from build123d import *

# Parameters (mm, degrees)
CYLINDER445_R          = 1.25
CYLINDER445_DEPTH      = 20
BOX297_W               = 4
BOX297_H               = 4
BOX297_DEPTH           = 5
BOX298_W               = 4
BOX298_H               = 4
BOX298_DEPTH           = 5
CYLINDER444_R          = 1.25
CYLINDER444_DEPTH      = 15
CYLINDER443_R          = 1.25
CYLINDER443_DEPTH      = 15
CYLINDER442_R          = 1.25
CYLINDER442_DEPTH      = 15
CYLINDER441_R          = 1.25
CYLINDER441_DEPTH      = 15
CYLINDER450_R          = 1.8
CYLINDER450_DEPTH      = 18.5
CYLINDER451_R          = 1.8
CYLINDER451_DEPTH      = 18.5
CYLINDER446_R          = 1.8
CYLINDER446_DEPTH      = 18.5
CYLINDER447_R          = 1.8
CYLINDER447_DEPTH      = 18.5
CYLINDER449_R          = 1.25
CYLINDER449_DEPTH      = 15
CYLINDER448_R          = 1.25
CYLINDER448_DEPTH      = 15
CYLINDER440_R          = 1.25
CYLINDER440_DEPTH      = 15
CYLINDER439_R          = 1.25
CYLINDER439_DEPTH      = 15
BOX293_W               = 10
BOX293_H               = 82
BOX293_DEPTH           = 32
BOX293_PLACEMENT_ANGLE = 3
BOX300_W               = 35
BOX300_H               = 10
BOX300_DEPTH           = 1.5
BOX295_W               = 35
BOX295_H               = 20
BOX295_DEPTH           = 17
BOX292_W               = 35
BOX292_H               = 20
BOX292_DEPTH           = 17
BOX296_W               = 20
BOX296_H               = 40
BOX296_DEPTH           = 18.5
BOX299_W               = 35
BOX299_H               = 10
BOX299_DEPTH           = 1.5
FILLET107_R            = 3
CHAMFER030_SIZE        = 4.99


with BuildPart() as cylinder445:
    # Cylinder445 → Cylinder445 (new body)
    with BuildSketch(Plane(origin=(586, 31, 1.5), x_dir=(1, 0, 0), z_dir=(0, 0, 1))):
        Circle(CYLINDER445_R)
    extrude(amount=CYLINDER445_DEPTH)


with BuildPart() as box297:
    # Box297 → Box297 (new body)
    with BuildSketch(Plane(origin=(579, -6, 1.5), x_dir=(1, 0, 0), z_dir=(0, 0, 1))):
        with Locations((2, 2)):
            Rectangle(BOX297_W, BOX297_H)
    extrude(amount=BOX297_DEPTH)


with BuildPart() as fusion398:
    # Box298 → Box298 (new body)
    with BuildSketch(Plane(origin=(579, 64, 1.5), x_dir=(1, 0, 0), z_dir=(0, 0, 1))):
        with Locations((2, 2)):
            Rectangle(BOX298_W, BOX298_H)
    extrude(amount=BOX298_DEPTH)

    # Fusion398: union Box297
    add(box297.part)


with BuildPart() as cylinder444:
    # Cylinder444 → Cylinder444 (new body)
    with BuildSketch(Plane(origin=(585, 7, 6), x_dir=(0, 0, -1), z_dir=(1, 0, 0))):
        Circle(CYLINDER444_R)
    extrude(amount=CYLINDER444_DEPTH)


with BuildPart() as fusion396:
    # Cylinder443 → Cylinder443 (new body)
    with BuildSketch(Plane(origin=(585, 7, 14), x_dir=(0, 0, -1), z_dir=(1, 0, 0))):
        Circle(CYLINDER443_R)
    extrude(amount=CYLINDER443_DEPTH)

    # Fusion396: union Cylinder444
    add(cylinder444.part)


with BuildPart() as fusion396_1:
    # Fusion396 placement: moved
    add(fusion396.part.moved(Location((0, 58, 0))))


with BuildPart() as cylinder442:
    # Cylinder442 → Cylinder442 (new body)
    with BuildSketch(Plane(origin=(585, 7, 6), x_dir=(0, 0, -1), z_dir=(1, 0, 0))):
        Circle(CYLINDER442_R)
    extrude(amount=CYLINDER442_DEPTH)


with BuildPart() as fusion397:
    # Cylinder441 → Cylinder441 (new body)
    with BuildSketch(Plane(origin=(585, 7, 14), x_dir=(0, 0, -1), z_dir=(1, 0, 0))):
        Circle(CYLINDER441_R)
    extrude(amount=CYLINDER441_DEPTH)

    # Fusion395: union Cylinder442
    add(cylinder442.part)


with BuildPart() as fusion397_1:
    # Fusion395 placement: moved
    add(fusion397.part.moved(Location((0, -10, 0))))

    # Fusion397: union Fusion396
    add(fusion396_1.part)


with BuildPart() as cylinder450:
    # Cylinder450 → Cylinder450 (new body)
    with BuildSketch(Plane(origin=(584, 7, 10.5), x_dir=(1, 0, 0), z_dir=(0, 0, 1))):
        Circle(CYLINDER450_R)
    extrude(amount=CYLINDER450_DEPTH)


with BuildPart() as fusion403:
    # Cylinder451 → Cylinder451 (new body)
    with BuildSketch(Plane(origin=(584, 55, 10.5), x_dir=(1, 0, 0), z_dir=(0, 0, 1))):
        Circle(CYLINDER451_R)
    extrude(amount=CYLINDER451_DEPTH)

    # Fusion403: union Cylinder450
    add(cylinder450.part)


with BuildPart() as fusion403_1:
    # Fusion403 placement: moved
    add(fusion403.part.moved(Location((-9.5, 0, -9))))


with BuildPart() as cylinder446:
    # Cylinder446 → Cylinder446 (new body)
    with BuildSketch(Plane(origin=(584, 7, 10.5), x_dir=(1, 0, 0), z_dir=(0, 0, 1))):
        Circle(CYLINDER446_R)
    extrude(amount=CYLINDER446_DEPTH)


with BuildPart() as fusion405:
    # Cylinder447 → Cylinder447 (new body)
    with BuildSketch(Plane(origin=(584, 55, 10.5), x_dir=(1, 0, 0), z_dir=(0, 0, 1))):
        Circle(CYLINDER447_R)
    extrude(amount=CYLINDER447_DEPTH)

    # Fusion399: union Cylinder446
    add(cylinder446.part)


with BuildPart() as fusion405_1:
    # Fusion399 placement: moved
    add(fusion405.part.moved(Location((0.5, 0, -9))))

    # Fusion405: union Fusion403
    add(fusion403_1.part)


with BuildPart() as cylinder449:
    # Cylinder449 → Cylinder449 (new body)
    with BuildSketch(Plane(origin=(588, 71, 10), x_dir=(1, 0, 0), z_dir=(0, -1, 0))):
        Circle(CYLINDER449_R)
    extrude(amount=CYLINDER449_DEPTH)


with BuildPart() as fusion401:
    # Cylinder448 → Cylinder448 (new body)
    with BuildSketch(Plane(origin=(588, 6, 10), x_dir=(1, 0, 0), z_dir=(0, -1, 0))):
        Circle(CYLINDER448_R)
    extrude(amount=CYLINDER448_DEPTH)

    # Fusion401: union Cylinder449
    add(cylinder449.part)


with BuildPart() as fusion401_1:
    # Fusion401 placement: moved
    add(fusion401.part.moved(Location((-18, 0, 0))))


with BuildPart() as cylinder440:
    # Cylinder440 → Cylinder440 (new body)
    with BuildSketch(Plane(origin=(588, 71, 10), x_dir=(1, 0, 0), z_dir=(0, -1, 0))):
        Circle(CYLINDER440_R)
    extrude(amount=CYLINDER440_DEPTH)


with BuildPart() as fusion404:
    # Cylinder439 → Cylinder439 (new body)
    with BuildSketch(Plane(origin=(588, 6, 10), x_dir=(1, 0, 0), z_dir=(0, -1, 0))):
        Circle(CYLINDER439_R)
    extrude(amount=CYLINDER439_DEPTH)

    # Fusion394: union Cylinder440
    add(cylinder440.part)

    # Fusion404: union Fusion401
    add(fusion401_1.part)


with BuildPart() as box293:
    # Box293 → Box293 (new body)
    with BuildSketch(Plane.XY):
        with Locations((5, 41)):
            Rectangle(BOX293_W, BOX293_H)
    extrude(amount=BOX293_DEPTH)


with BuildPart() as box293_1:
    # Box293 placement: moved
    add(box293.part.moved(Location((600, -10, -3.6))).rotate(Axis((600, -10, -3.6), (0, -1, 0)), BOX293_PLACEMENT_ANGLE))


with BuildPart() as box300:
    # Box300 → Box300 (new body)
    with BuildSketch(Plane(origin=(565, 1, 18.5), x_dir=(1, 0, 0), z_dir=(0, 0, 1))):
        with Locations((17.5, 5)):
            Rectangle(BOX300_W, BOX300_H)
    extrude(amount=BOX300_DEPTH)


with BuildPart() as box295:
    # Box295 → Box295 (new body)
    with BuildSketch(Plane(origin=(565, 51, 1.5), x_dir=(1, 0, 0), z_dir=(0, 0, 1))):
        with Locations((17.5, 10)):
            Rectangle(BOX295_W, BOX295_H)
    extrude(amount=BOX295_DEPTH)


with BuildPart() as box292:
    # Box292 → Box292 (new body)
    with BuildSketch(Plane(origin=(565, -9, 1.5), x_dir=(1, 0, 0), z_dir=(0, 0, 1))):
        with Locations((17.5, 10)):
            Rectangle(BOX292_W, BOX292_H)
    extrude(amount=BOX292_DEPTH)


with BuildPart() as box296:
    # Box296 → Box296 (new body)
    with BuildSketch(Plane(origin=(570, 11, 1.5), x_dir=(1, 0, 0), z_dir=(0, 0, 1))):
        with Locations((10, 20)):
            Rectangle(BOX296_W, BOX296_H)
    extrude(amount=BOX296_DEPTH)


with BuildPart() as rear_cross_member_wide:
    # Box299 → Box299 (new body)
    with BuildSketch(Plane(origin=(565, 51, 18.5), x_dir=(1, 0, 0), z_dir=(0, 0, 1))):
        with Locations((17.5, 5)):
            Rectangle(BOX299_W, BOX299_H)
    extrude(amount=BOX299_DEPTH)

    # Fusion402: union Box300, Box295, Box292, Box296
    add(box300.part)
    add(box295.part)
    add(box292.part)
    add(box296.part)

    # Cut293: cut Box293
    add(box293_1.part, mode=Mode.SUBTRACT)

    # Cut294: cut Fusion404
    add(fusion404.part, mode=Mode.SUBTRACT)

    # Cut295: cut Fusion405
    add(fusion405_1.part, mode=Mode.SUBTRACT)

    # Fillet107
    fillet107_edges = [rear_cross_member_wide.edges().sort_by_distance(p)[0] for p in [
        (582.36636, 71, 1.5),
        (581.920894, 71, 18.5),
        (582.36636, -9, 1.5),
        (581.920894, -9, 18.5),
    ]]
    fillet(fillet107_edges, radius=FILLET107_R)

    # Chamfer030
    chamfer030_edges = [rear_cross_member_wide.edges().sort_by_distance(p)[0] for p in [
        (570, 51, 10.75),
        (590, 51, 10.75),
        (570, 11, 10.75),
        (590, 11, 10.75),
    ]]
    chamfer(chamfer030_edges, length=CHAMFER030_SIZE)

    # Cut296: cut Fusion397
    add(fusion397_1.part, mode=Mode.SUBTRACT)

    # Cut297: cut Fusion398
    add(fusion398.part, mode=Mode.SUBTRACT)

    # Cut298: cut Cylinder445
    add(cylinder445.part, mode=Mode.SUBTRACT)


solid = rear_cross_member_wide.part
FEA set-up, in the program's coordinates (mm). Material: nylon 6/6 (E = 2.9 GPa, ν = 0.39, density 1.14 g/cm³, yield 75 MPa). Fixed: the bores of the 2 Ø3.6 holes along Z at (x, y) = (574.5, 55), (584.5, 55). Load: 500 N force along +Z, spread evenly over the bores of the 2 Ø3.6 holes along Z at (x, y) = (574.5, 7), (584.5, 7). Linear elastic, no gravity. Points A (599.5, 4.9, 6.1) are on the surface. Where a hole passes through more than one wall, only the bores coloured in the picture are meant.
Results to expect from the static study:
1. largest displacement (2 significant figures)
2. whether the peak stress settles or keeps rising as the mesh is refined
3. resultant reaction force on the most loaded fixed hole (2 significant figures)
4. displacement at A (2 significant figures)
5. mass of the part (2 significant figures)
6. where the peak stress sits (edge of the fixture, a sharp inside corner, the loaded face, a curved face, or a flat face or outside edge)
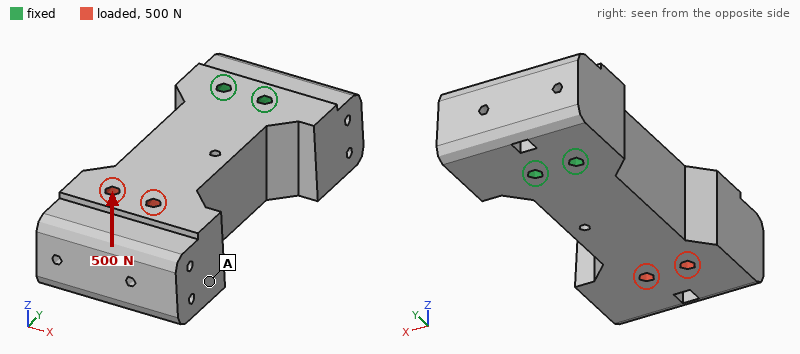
0.93 mm
keeps rising
250 N
0.66 mm
44 g
edge of the fixture
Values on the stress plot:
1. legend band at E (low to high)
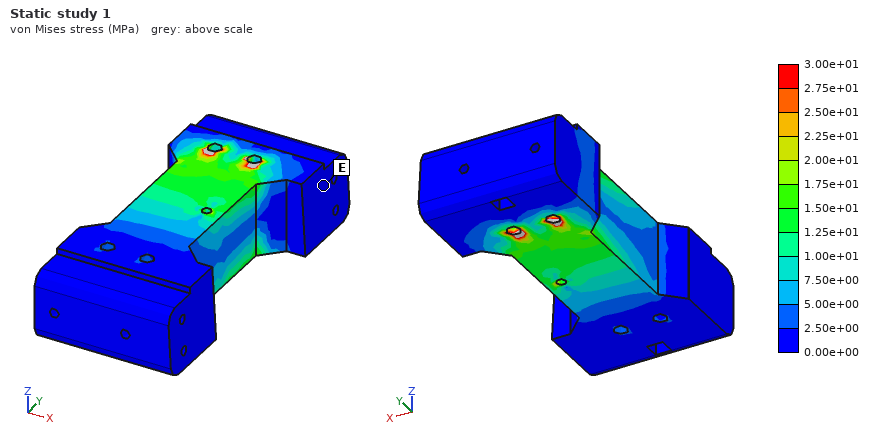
0.00e+00 to 2.50e+00 MPa
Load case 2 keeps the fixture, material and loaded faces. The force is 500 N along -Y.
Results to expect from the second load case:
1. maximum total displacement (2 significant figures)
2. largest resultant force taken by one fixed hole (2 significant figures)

26 µm
260 N
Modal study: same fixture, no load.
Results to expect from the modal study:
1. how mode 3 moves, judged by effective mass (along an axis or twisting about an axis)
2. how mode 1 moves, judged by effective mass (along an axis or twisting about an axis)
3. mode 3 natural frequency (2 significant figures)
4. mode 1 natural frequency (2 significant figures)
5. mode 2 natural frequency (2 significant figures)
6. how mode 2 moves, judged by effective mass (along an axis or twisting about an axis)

twisting about Y
along Z
2400 Hz
950 Hz
990 Hz
along X
